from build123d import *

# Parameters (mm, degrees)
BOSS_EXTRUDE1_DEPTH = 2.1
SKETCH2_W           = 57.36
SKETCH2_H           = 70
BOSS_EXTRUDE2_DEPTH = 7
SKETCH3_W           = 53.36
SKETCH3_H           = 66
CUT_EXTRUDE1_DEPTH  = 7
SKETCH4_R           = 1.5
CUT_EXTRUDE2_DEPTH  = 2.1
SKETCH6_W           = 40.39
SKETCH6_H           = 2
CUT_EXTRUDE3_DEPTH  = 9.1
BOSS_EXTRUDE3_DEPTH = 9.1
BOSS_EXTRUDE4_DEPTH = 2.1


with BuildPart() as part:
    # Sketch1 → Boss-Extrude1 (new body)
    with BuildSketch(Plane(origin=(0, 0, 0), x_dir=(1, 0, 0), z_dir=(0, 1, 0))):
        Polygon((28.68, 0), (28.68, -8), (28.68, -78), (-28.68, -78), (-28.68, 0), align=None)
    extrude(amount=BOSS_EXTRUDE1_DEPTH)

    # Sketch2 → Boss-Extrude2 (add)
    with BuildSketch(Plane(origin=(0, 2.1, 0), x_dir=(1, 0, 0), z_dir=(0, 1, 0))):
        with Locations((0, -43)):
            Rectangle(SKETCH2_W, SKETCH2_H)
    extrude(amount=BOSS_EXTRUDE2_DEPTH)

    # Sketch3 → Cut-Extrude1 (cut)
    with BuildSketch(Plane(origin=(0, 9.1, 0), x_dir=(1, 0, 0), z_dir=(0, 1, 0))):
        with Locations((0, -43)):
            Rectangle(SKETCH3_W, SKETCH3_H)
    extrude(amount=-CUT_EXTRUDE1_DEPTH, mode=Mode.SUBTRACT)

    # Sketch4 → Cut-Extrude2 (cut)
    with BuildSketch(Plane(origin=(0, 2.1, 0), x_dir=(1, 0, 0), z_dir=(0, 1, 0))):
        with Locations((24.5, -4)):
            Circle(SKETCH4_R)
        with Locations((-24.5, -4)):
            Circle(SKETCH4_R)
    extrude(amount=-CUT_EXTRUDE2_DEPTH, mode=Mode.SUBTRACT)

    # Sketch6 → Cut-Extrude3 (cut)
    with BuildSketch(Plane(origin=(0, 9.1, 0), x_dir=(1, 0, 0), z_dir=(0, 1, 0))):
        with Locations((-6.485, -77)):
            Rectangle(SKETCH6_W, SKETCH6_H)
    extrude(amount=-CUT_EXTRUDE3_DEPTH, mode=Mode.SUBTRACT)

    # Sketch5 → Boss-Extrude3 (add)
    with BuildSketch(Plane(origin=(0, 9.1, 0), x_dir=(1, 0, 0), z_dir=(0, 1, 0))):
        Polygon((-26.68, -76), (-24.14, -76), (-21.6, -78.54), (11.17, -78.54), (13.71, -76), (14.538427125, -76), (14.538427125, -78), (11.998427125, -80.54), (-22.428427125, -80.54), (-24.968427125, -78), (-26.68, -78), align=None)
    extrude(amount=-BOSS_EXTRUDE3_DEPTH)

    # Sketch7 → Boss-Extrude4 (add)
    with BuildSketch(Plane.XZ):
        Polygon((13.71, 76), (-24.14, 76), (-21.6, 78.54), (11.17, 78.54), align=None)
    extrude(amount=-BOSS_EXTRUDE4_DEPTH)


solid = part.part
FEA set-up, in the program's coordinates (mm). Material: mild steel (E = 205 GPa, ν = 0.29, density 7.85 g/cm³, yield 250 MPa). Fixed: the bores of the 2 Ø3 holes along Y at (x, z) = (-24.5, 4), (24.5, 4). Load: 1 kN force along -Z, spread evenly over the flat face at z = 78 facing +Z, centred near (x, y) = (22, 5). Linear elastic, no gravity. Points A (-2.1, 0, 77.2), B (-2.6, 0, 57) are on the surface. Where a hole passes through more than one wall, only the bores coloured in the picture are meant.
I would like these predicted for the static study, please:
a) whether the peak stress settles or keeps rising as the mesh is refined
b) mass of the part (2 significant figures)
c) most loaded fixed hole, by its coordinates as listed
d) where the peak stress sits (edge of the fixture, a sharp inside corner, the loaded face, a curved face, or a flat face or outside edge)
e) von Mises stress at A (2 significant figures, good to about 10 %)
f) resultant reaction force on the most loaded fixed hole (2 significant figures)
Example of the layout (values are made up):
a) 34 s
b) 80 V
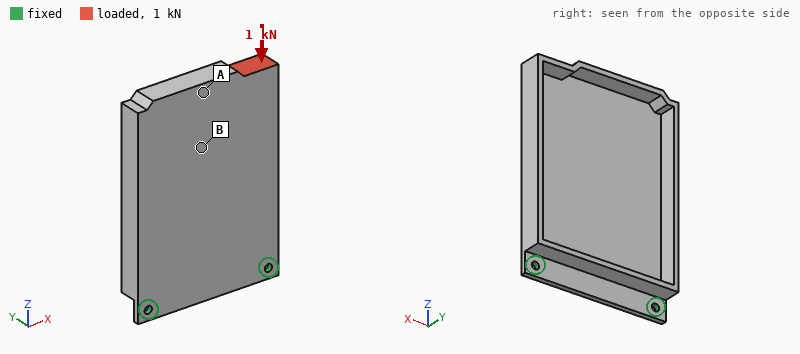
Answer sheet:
a) keeps rising
b) 100 g
c) (24.5, 4)
d) edge of the fixture
e) 31 MPa
f) 940 N
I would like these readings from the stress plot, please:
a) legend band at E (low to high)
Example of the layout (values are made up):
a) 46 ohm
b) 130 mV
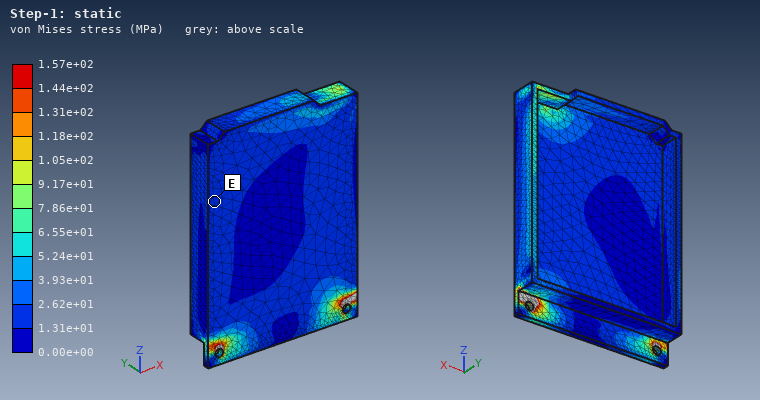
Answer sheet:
a) 1.31e+01 to 2.62e+01 MPa
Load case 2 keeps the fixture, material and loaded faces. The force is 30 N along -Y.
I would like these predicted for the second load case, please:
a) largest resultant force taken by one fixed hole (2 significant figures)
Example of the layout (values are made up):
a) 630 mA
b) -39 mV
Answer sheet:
a) 73 N
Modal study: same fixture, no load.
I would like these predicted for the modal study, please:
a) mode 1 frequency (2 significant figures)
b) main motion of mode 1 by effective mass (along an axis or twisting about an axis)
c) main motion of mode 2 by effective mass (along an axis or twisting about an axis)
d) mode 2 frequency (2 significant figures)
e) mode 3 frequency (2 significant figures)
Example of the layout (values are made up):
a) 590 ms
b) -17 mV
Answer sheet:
a) 320 Hz
b) along Y
c) twisting about Z
d) 890 Hz
e) 3100 Hz
